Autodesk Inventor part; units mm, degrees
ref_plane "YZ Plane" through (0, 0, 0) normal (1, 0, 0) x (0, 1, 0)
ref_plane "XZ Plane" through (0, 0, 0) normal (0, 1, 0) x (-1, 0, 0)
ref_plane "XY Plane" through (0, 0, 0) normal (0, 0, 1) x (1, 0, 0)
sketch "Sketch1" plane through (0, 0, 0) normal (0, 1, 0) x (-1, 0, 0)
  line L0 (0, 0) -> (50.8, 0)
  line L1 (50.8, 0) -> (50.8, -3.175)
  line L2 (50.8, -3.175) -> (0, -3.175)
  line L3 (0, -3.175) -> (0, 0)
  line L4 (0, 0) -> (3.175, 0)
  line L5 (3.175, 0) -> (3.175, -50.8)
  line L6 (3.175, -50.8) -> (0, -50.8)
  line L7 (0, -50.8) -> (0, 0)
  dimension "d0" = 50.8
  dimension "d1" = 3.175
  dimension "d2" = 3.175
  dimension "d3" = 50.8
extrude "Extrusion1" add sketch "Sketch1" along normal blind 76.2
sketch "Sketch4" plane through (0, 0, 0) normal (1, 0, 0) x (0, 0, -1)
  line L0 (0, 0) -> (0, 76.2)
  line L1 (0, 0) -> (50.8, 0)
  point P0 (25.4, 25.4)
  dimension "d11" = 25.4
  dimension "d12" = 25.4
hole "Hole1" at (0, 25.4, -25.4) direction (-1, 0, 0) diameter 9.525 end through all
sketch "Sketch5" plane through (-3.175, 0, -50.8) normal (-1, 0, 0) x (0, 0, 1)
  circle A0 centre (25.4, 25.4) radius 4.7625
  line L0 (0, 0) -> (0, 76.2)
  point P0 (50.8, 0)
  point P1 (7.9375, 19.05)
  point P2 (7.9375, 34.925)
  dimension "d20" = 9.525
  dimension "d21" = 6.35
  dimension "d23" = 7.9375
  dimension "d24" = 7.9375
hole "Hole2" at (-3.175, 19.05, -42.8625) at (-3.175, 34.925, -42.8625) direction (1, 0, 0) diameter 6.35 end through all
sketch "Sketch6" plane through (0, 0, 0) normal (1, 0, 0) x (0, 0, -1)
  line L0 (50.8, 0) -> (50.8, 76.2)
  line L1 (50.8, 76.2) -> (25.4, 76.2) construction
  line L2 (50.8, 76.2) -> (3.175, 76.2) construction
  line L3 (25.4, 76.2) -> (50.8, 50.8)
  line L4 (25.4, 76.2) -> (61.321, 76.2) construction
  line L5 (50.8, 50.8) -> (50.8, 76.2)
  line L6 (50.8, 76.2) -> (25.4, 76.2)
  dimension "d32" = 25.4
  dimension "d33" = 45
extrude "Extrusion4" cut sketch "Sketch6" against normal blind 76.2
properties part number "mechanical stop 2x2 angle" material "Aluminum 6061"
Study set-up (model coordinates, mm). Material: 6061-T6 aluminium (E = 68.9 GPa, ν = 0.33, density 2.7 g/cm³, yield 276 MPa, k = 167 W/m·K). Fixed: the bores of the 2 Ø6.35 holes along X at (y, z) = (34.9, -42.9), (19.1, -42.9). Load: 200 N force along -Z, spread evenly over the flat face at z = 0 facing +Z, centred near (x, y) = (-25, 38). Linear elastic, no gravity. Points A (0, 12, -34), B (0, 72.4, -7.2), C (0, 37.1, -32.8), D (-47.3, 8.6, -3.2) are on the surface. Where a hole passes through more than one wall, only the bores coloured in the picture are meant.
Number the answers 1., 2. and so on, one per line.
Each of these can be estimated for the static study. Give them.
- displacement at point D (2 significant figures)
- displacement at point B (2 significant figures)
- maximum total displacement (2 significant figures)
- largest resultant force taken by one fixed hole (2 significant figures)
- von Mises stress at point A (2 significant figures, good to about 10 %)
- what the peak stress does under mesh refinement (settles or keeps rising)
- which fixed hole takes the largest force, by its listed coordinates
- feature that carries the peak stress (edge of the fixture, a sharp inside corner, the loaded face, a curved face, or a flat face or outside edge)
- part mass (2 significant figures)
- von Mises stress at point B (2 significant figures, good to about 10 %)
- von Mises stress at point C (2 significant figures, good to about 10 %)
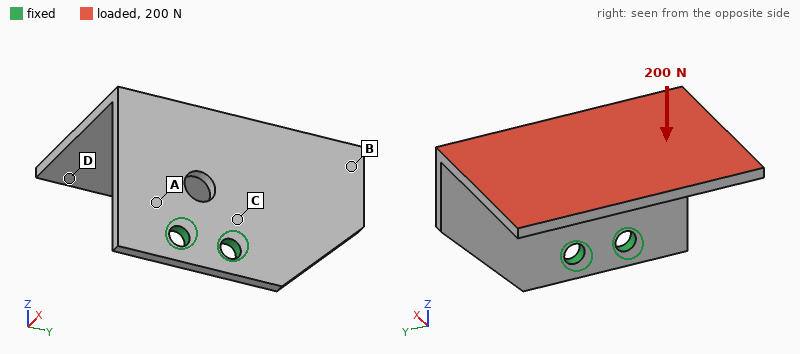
1. 0.93 mm
2. 0.31 mm
3. 1.1 mm
4. 200 N
5. 43 MPa
6. keeps rising
7. (34.9, -42.9)
8. edge of the fixture
9. 60 g
10. 30 MPa
11. 48 MPa
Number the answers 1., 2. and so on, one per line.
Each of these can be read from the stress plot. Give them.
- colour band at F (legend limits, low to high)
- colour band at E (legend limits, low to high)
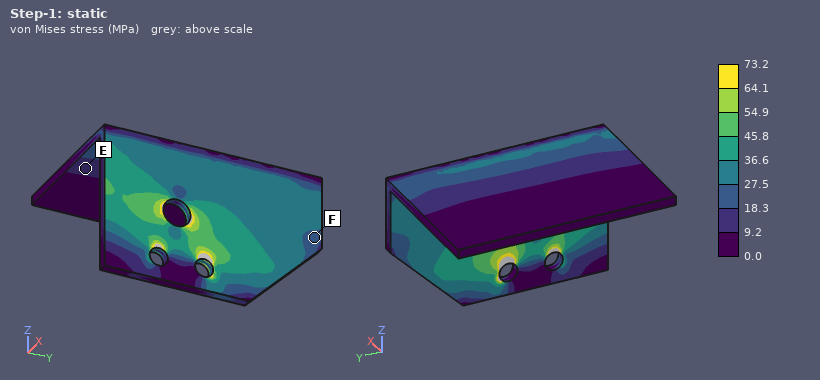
1. 18.3 to 27.5 MPa
2. 9.2 to 18.3 MPa
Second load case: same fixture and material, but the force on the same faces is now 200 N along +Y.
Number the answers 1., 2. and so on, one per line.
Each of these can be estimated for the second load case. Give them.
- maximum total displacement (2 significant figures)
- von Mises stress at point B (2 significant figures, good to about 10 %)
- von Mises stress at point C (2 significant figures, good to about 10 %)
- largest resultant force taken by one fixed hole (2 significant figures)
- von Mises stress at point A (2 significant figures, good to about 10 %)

1. 0.54 mm
2. 12 MPa
3. 35 MPa
4. 400 N
5. 30 MPa
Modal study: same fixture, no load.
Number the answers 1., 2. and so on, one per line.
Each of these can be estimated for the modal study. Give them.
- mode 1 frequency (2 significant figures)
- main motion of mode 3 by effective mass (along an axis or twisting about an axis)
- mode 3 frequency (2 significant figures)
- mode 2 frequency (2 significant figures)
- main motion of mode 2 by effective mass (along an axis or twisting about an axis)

1. 380 Hz
2. along X
3. 1100 Hz
4. 580 Hz
5. along Y
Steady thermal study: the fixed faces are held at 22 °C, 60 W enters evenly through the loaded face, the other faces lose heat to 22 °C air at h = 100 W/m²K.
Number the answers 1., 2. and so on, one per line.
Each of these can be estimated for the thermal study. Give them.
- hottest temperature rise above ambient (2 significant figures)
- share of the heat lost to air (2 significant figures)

1. 58 K
2. 60 %
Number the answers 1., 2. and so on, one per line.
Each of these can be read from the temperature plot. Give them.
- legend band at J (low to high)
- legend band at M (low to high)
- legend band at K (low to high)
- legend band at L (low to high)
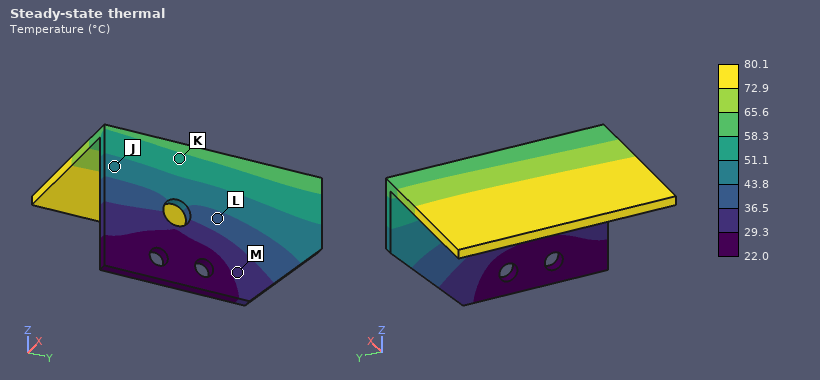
1. 43.8 to 51.1 °C
2. 29.3 to 36.5 °C
3. 51.1 to 58.3 °C
4. 36.5 to 43.8 °C
